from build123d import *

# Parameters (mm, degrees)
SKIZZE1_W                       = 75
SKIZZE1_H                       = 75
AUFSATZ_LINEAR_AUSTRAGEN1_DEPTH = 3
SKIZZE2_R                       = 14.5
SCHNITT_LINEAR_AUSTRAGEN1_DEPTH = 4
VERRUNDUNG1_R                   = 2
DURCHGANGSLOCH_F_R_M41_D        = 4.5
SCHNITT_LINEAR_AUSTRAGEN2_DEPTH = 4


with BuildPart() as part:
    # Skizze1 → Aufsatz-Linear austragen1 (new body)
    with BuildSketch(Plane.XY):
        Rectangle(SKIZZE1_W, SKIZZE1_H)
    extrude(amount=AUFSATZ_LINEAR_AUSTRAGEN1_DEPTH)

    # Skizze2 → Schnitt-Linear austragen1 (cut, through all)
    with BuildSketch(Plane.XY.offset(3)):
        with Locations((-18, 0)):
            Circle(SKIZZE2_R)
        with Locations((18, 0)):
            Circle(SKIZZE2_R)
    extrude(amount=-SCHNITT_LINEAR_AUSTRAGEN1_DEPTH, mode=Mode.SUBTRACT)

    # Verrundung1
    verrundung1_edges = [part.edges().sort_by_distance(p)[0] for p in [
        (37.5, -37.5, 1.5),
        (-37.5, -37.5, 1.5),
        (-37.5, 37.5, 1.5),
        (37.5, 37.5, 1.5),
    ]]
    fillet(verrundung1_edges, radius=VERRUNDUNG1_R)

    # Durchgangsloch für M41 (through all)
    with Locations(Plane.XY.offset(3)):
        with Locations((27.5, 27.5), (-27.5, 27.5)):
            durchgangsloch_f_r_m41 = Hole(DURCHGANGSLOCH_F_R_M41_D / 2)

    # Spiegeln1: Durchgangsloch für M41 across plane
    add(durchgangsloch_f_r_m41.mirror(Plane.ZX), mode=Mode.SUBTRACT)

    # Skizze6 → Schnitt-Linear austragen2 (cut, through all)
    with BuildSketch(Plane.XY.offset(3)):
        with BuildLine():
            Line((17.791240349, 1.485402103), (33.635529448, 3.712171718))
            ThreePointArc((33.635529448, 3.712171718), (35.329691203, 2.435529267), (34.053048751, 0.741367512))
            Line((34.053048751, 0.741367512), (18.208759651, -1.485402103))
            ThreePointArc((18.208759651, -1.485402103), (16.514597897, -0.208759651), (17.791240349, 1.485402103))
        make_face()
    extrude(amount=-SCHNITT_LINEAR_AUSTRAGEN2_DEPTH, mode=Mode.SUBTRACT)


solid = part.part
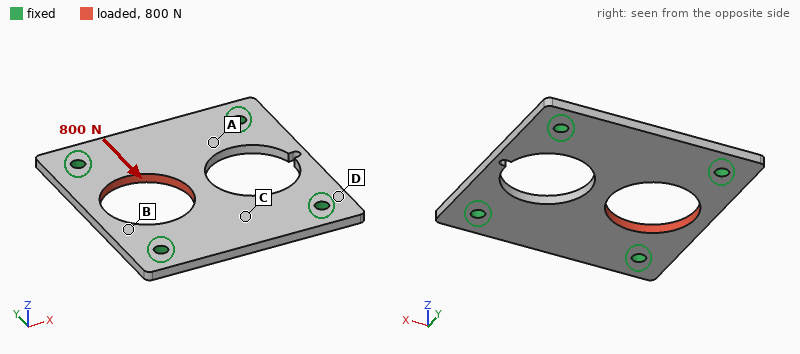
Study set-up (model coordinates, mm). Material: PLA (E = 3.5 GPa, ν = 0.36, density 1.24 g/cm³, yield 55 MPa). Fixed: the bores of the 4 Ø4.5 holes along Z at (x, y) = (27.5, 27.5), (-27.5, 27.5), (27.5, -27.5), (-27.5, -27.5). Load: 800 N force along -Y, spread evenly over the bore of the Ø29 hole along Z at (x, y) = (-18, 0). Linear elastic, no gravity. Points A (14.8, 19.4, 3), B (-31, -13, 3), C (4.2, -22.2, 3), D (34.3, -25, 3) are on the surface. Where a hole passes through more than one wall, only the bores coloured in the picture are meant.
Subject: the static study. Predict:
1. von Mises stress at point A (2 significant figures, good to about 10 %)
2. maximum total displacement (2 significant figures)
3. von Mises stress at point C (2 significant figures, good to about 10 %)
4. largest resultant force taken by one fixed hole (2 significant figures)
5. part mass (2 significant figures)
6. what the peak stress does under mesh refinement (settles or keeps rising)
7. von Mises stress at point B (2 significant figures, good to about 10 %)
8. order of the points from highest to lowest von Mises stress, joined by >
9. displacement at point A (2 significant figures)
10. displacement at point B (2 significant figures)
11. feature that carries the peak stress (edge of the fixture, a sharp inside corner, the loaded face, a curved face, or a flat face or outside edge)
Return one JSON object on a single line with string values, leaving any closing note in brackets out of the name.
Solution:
{"von Mises stress at point A": "3.0 MPa", "maximum total displacement": "53 µm", "von Mises stress at point C": "1.8 MPa", "largest resultant force taken by one fixed hole": "320 N", "part mass": "16 g", "what the peak stress does under mesh refinement": "keeps rising", "von Mises stress at point B": "4.5 MPa", "order of the points from highest to lowest von Mises stress, joined by >": "B > A > C > D", "displacement at point A": "25 µm", "displacement at point B": "20 µm", "feature that carries the peak stress": "edge of the fixture"}
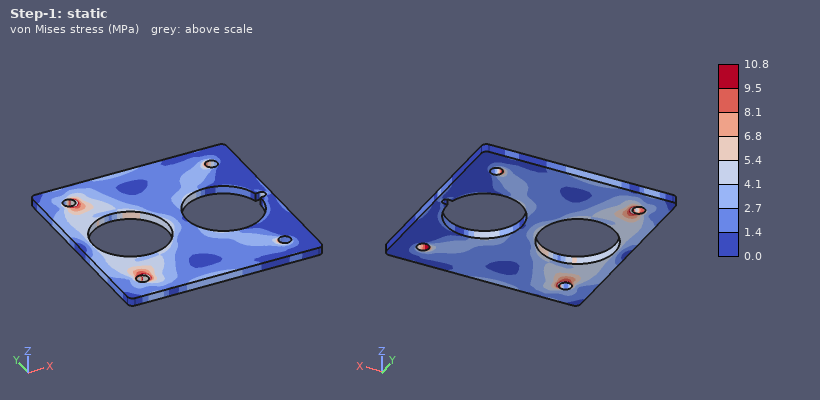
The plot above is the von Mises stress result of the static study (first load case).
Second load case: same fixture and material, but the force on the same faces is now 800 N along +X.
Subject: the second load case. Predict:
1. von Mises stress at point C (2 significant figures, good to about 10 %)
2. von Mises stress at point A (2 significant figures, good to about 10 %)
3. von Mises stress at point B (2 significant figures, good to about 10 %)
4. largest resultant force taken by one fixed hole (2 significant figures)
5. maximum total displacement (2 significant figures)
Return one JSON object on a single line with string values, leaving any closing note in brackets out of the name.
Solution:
{"von Mises stress at point C": "2.3 MPa", "von Mises stress at point A": "3.9 MPa", "von Mises stress at point B": "6.7 MPa", "largest resultant force taken by one fixed hole": "250 N", "maximum total displacement": "0.15 mm"}
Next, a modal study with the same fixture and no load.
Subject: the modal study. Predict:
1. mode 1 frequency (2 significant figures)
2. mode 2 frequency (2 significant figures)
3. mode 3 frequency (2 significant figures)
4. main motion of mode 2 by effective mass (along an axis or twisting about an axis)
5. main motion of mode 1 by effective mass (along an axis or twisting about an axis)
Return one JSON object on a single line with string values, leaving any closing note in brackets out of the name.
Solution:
{"mode 1 frequency": "1300 Hz", "mode 2 frequency": "1800 Hz", "mode 3 frequency": "2000 Hz", "main motion of mode 2 by effective mass": "twisting about X", "main motion of mode 1 by effective mass": "along Z"}
